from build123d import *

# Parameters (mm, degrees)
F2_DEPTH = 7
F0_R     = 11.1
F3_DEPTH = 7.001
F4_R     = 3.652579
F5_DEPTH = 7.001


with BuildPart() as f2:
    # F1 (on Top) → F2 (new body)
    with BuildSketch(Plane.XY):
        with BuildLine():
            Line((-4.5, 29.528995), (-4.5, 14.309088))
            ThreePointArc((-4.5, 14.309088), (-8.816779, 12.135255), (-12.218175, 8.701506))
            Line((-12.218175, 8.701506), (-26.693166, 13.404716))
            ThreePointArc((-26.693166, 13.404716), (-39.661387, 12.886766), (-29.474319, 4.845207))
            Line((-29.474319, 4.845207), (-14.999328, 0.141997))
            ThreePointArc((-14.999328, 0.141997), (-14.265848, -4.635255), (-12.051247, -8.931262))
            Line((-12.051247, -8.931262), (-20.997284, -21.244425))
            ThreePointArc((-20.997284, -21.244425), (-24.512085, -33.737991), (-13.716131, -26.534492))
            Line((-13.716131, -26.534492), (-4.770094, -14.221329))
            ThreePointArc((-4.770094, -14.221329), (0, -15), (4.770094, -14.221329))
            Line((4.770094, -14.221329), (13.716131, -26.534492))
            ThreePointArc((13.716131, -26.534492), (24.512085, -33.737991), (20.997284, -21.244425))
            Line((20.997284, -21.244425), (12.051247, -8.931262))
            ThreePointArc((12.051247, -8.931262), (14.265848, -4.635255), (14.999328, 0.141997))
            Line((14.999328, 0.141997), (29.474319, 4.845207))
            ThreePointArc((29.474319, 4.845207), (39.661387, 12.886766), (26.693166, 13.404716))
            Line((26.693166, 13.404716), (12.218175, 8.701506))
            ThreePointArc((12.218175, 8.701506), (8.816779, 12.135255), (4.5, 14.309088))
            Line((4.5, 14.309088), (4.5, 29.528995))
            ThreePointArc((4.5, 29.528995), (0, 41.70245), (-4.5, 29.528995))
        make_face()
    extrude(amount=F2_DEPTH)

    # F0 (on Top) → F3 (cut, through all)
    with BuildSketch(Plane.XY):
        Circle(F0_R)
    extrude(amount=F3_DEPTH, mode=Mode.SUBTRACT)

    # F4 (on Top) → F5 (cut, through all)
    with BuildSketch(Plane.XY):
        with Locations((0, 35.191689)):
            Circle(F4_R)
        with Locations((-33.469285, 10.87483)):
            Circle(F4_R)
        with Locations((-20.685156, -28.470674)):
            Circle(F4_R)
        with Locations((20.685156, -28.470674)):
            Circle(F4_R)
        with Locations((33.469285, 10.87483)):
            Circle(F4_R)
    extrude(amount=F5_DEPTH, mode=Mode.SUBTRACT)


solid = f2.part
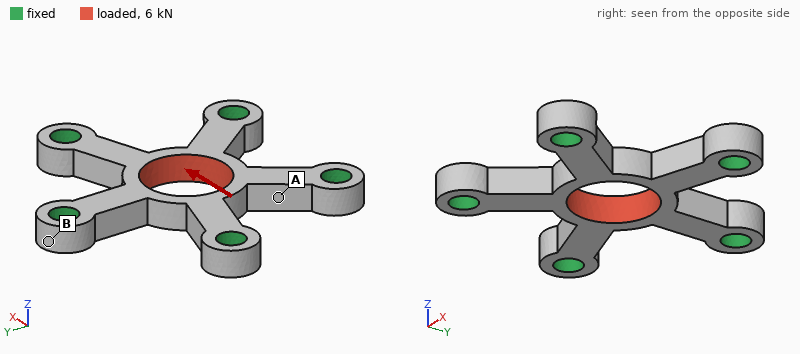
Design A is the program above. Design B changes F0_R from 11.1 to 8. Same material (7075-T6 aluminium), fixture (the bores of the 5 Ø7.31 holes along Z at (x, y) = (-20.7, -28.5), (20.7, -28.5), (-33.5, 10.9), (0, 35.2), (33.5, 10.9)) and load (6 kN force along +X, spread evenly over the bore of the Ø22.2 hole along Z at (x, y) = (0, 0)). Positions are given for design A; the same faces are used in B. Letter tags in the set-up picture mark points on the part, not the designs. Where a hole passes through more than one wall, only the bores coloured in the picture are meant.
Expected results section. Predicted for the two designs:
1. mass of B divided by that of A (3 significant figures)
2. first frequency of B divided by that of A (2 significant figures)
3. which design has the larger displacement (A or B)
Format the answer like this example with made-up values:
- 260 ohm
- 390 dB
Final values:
- 1.13
- 0.89
- A
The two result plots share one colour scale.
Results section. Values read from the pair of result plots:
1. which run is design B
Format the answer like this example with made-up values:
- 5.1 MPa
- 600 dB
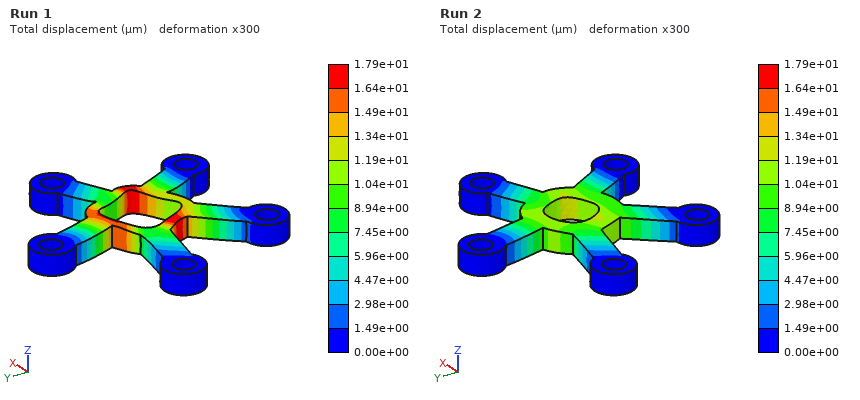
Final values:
- Run 2
